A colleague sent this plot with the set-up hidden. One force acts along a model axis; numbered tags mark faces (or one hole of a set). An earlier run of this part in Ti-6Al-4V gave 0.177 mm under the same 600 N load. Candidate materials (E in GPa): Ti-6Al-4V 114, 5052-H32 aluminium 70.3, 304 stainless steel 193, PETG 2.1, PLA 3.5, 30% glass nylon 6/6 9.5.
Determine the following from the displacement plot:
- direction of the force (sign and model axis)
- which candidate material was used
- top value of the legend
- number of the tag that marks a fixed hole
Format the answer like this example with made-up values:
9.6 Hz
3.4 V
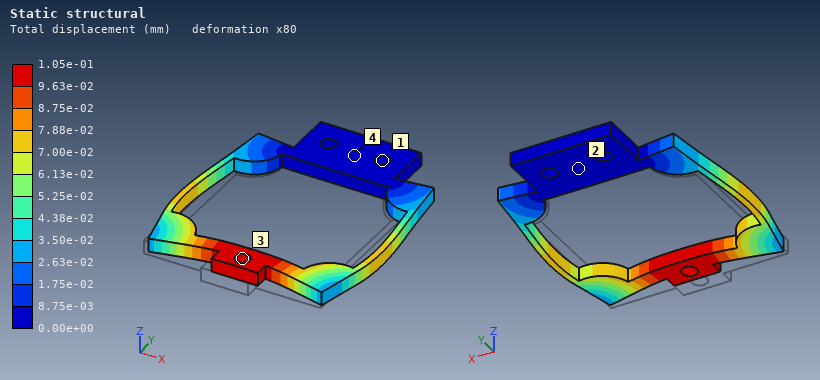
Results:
+Y
304 stainless steel
1.05e-01 mm
1
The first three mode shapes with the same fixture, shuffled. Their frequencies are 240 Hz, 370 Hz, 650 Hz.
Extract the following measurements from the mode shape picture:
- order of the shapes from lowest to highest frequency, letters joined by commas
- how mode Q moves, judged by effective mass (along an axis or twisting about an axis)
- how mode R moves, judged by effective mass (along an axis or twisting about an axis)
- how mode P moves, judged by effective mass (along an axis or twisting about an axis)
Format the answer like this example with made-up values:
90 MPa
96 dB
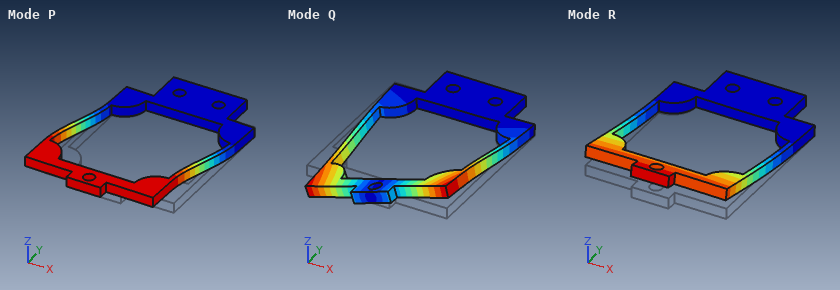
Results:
R, P, Q
twisting about Y
along Z
along X
